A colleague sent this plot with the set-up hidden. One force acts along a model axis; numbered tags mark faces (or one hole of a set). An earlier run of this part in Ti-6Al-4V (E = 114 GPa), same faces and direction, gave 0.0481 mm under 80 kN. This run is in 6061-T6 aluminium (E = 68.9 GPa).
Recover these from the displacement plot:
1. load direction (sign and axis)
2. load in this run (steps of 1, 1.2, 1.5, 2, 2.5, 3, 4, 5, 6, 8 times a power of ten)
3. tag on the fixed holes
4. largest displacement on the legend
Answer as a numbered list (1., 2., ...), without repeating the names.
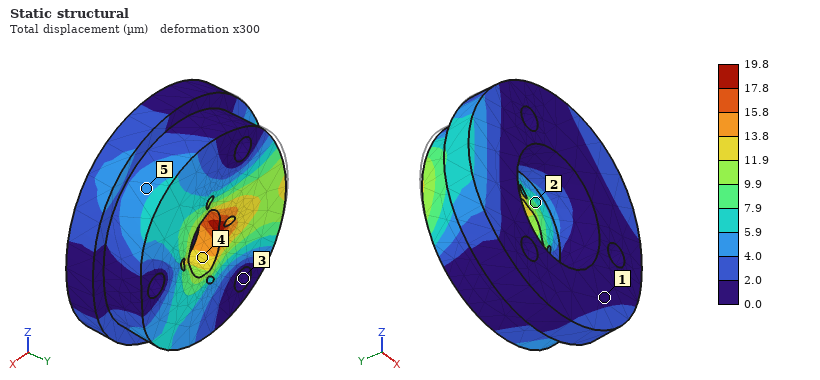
1. +X
2. 20 kN
3. 3
4. 19.8 µm
